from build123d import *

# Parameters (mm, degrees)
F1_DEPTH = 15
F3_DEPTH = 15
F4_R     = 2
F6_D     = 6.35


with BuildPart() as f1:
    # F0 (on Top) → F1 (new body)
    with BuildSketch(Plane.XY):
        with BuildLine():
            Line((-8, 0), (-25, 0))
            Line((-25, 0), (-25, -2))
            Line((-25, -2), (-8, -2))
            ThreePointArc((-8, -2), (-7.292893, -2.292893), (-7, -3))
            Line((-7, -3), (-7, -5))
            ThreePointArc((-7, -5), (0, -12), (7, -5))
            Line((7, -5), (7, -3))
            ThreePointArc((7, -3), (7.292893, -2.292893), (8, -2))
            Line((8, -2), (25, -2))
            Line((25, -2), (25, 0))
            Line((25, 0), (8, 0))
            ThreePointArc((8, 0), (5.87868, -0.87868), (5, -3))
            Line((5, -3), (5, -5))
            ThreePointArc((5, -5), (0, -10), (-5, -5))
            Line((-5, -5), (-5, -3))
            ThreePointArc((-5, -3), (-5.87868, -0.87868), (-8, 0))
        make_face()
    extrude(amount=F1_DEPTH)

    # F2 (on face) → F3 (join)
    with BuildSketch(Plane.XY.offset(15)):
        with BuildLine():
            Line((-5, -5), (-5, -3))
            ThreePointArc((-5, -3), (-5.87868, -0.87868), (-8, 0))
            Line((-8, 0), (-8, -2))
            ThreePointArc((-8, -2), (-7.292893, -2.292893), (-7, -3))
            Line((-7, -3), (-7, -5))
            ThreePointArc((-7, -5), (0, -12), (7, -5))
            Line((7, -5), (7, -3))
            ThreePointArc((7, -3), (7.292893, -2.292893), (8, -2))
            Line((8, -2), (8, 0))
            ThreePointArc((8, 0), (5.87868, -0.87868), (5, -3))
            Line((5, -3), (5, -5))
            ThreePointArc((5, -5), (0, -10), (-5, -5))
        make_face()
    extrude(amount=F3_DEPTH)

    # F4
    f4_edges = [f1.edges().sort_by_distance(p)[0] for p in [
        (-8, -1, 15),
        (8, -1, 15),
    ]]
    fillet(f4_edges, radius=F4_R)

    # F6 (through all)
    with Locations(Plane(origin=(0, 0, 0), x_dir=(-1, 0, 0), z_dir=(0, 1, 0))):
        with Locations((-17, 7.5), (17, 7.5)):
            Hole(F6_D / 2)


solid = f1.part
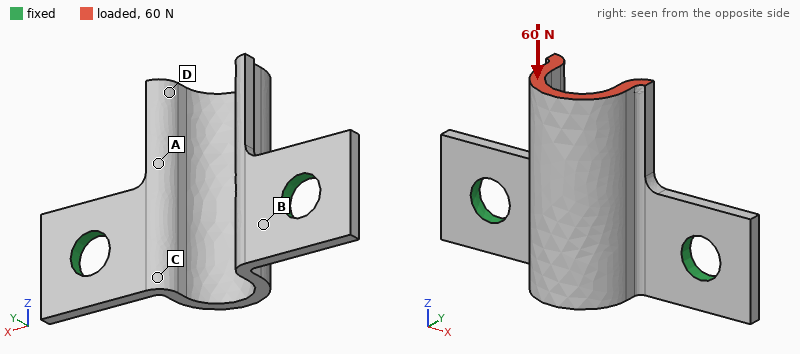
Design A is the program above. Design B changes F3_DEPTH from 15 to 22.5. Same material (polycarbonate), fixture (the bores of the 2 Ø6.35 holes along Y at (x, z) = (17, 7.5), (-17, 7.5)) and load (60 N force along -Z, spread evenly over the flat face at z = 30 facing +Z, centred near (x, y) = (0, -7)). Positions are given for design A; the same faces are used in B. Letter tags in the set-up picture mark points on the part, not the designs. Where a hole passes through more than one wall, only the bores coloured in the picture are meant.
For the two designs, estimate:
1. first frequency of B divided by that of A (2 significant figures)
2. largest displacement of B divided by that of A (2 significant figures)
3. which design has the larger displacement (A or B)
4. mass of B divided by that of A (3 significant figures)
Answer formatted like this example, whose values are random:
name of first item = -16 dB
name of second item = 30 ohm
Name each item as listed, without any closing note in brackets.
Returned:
first frequency of B divided by that of A = 0.70
largest displacement of B divided by that of A = 1.3
which design has the larger displacement = B
mass of B divided by that of A = 1.17
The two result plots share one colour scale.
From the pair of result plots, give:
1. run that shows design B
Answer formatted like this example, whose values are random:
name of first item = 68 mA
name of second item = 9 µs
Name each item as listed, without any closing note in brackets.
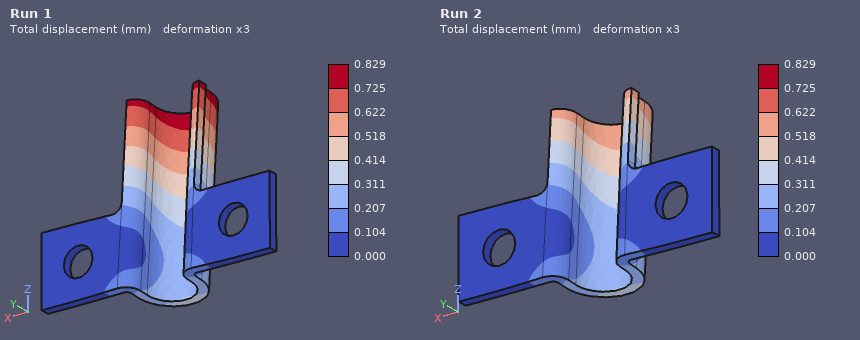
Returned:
run that shows design B = Run 1
